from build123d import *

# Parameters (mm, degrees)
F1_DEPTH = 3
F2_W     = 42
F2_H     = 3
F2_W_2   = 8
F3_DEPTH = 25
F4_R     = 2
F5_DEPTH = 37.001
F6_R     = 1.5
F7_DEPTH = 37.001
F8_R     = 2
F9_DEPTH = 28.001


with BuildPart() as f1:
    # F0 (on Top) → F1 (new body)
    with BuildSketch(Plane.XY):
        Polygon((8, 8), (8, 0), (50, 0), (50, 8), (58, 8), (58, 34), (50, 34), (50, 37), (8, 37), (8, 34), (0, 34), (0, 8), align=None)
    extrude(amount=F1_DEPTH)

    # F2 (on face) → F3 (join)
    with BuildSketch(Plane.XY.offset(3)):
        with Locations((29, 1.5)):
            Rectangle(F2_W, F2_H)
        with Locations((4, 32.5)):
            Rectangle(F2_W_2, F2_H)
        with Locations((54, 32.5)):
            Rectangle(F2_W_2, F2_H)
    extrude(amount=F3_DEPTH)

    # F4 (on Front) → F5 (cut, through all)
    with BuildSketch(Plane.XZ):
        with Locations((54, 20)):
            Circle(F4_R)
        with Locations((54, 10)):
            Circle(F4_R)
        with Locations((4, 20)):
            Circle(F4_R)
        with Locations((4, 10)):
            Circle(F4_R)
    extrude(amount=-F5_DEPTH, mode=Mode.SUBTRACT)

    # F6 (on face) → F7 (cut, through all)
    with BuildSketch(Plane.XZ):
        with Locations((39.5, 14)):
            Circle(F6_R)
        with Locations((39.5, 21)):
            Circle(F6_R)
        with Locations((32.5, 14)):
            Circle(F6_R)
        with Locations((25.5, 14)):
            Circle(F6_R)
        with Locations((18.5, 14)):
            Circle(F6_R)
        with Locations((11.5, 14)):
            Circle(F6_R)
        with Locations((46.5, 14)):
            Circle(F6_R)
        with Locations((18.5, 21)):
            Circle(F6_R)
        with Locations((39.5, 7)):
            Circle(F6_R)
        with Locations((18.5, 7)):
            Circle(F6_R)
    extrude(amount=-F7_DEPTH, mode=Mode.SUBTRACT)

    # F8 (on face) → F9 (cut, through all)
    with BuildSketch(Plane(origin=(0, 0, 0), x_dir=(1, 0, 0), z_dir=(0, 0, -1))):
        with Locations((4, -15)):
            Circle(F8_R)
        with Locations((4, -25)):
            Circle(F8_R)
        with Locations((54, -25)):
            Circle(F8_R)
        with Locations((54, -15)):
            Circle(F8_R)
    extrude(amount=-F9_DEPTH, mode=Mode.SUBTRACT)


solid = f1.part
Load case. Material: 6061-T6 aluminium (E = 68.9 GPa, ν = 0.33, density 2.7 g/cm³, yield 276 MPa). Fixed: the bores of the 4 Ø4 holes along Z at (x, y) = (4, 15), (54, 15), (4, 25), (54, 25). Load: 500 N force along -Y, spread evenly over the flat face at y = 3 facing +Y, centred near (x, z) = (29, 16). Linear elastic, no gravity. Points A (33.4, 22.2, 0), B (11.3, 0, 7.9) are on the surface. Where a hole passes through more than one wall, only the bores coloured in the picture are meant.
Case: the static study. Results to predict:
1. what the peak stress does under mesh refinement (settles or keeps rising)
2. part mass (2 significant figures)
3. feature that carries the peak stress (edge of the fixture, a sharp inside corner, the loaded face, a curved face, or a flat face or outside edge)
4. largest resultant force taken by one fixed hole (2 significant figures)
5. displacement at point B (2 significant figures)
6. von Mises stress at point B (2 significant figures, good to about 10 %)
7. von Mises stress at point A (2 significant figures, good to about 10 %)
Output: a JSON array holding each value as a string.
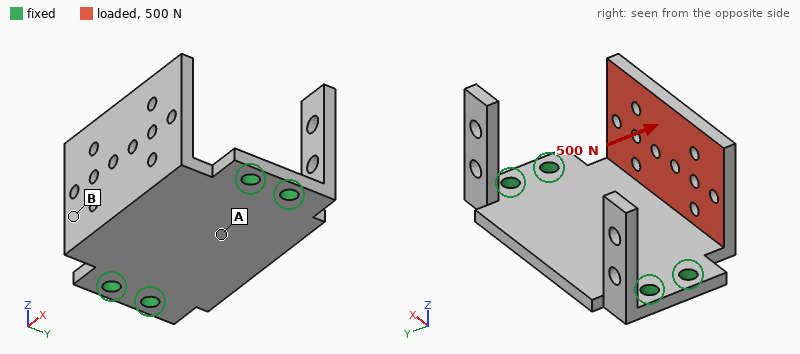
["keeps rising", "26 g", "edge of the fixture", "230 N", "0.19 mm", "66 MPa", "26 MPa"]
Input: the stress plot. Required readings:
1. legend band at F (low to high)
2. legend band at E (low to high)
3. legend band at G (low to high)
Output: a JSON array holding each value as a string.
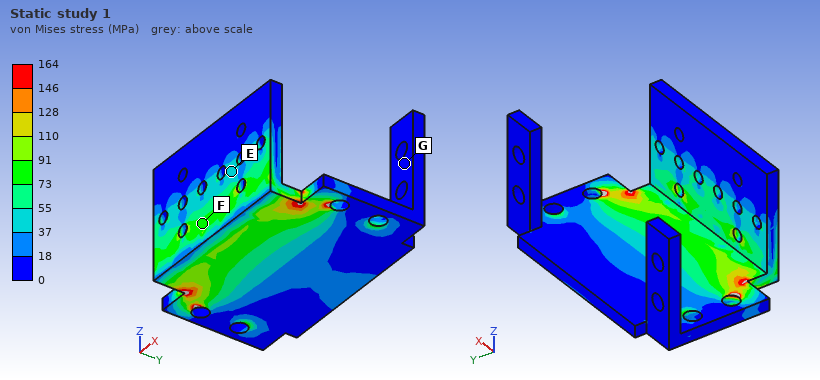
["73 to 91 MPa", "37 to 55 MPa", "0 to 18 MPa"]
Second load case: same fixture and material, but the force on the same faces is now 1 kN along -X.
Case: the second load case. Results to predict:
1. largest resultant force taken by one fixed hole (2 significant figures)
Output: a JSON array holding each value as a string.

["580 N"]
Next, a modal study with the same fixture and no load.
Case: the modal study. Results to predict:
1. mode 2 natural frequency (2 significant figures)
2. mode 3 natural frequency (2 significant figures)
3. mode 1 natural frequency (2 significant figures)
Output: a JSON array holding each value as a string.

["2800 Hz", "2800 Hz", "1900 Hz"]
